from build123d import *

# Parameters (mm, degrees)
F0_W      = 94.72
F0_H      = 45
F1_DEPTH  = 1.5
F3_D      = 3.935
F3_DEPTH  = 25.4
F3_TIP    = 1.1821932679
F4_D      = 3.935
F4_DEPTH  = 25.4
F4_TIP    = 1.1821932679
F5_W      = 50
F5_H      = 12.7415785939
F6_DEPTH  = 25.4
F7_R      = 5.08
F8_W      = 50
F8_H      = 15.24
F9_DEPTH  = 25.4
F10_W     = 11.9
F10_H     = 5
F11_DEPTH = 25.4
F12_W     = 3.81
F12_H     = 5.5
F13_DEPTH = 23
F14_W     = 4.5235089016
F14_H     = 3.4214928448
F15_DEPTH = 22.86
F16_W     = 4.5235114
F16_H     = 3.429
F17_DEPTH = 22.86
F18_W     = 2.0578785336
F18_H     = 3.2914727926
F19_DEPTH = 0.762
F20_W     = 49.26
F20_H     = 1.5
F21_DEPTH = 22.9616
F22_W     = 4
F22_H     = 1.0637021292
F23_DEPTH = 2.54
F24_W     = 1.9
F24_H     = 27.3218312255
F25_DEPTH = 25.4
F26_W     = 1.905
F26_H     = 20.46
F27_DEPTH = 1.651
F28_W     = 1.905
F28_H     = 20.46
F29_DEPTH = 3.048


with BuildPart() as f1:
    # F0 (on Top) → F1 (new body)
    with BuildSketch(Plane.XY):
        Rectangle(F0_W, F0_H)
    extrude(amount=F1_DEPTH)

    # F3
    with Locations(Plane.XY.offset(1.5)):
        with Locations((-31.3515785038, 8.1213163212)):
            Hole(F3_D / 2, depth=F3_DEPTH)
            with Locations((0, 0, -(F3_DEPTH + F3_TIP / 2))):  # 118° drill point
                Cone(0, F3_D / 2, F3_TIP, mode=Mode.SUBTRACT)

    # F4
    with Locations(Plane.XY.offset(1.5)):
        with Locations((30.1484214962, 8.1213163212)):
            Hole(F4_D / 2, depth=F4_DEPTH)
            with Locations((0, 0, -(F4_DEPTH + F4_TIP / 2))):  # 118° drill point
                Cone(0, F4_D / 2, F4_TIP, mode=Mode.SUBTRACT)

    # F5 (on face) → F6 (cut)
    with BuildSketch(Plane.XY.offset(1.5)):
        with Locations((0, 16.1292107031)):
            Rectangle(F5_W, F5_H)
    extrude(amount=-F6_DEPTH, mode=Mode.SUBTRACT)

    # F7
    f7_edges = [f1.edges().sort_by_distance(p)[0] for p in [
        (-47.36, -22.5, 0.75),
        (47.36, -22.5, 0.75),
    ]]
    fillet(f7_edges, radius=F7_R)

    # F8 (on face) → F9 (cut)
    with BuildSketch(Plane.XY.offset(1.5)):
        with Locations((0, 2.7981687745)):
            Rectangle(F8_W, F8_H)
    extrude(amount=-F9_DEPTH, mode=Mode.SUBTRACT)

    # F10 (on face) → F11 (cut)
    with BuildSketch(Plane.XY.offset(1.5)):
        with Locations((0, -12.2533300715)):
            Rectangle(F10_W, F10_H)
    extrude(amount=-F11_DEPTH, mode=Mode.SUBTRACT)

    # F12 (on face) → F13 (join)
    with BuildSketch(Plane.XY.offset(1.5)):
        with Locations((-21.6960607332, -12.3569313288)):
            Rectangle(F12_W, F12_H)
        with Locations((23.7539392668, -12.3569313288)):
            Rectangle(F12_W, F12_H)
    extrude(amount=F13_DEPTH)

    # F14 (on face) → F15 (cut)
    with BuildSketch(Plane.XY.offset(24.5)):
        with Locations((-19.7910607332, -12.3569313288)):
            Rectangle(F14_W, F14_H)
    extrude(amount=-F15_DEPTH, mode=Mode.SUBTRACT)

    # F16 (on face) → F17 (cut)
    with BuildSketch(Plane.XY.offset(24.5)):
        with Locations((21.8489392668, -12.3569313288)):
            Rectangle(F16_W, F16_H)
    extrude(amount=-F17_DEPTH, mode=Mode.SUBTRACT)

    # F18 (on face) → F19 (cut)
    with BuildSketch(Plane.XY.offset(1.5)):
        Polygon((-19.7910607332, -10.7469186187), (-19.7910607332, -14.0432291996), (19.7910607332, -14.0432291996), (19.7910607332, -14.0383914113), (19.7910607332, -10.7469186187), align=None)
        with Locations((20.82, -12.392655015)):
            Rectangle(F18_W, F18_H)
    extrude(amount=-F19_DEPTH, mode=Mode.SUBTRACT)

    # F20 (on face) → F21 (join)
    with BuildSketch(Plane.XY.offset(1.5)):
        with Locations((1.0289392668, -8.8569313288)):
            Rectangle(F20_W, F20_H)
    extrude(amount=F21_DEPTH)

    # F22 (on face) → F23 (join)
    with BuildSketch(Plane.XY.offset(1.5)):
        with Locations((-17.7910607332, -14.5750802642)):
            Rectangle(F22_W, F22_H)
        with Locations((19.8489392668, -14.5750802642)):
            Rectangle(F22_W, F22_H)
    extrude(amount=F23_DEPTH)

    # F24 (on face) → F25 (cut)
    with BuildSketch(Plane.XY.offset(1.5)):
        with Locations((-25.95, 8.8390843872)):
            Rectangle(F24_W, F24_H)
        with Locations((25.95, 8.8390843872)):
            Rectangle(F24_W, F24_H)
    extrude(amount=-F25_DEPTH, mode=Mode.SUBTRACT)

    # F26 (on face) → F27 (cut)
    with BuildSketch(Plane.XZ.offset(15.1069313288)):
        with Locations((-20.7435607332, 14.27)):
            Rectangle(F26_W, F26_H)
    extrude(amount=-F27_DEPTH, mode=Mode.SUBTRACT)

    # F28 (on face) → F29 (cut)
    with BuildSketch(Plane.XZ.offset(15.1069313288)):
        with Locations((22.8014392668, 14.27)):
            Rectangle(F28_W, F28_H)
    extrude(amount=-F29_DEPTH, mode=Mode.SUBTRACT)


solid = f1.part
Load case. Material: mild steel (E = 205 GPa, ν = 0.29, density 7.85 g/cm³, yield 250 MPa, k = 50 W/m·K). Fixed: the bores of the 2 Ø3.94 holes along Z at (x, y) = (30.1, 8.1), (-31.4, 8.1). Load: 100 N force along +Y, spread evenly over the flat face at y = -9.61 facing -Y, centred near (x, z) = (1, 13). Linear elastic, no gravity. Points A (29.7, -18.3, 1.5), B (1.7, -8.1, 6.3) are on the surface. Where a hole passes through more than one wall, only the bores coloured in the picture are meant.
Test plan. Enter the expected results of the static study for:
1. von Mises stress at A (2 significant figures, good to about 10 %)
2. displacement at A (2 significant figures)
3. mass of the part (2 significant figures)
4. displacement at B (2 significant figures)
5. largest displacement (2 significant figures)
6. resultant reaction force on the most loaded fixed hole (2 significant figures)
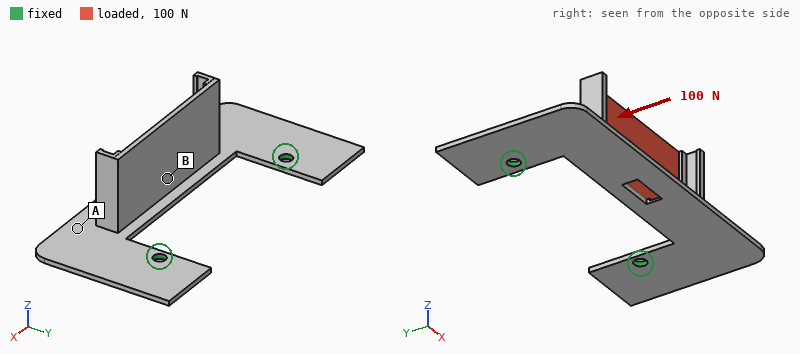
24 MPa
0.19 mm
49 g
0.10 mm
0.34 mm
58 N
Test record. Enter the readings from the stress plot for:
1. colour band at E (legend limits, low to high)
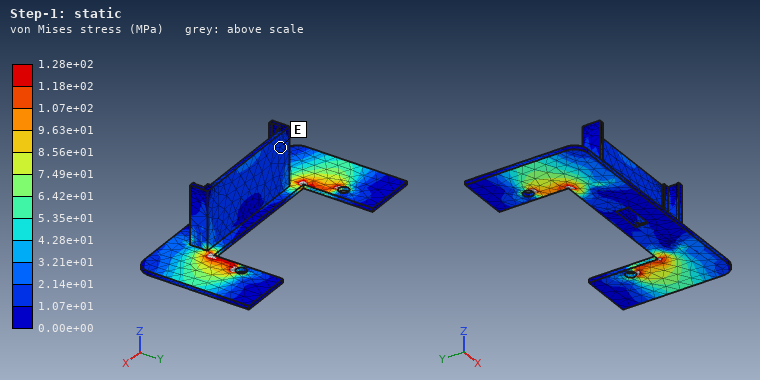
1.07e+01 to 2.14e+01 MPa
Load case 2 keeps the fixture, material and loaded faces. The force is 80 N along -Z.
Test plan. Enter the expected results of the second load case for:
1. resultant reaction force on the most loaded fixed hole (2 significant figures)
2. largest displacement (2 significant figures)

42 N
0.17 mm
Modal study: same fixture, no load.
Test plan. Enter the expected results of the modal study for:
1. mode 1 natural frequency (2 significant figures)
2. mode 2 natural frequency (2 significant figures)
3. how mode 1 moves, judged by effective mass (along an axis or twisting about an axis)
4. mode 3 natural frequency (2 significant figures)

570 Hz
1300 Hz
along Z
1700 Hz
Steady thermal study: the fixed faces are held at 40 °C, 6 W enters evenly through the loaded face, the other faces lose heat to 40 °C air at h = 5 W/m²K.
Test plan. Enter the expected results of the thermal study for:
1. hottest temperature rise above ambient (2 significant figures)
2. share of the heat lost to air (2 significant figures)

73 K
25 %
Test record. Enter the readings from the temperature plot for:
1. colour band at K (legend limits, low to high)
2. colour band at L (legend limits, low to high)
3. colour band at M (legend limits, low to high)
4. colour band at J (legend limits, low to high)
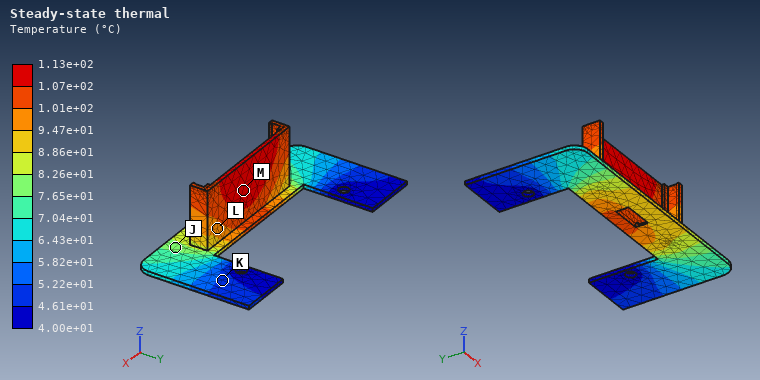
4.61e+01 to 5.22e+01 °C
9.47e+01 to 1.01e+02 °C
1.07e+02 to 1.13e+02 °C
7.65e+01 to 8.26e+01 °C
